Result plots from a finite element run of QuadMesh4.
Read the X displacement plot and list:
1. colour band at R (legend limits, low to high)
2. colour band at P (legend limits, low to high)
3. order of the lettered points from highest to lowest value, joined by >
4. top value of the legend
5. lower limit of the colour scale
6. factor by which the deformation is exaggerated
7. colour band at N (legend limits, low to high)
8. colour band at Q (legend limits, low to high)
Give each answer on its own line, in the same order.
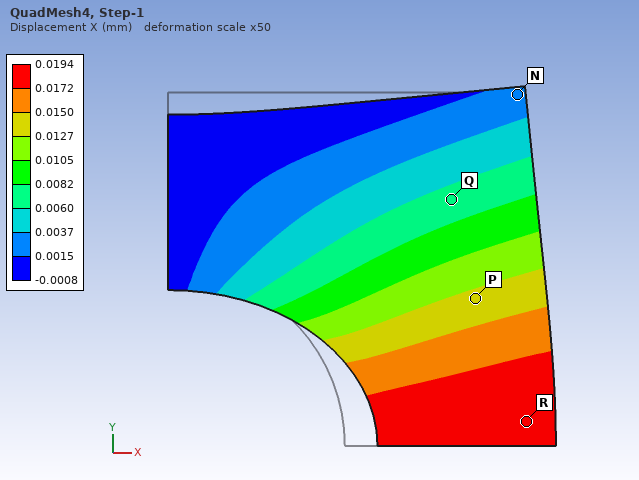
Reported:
0.0172 to 0.0194 mm
0.0127 to 0.0150 mm
R > P > Q > N
0.0194 mm
-0.0008 mm
50
0.0015 to 0.0037 mm
0.0060 to 0.0082 mm
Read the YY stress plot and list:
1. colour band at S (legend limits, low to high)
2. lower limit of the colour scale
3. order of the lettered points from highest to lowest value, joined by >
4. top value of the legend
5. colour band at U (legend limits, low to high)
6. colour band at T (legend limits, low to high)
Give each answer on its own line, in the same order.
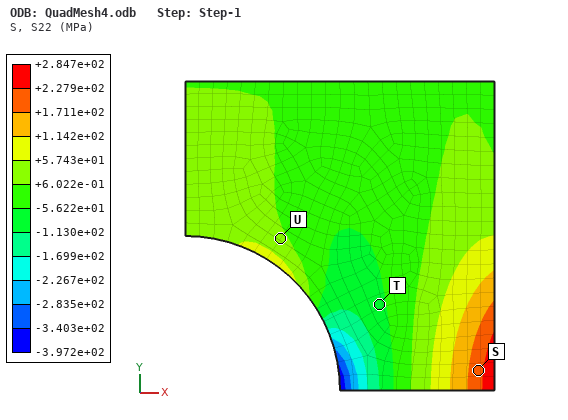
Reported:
+1.711e+02 to +2.279e+02 MPa
-3.972e+02 MPa
S > U > T
+2.847e+02 MPa
+6.022e-01 to +5.743e+01 MPa
-1.130e+02 to -5.622e+01 MPa
